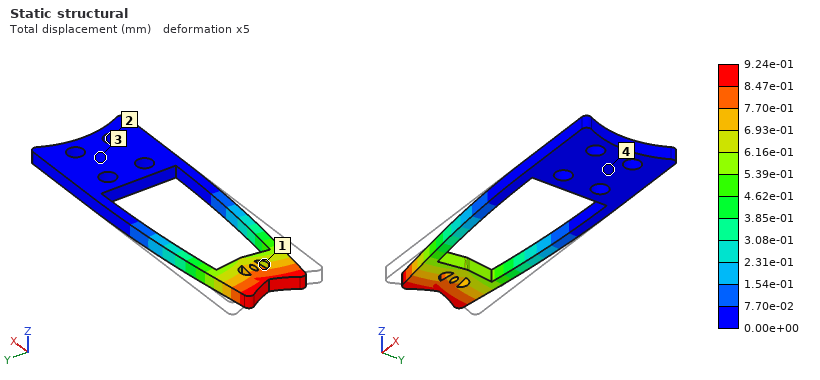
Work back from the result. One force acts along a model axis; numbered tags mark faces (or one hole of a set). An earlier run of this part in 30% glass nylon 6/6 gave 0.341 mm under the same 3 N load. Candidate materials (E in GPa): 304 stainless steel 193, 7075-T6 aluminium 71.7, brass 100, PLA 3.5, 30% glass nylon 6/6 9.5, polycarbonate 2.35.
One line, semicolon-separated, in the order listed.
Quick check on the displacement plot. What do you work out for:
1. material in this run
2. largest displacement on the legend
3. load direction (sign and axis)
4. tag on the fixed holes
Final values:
PLA; 9.24e-01 mm; +X; 2
